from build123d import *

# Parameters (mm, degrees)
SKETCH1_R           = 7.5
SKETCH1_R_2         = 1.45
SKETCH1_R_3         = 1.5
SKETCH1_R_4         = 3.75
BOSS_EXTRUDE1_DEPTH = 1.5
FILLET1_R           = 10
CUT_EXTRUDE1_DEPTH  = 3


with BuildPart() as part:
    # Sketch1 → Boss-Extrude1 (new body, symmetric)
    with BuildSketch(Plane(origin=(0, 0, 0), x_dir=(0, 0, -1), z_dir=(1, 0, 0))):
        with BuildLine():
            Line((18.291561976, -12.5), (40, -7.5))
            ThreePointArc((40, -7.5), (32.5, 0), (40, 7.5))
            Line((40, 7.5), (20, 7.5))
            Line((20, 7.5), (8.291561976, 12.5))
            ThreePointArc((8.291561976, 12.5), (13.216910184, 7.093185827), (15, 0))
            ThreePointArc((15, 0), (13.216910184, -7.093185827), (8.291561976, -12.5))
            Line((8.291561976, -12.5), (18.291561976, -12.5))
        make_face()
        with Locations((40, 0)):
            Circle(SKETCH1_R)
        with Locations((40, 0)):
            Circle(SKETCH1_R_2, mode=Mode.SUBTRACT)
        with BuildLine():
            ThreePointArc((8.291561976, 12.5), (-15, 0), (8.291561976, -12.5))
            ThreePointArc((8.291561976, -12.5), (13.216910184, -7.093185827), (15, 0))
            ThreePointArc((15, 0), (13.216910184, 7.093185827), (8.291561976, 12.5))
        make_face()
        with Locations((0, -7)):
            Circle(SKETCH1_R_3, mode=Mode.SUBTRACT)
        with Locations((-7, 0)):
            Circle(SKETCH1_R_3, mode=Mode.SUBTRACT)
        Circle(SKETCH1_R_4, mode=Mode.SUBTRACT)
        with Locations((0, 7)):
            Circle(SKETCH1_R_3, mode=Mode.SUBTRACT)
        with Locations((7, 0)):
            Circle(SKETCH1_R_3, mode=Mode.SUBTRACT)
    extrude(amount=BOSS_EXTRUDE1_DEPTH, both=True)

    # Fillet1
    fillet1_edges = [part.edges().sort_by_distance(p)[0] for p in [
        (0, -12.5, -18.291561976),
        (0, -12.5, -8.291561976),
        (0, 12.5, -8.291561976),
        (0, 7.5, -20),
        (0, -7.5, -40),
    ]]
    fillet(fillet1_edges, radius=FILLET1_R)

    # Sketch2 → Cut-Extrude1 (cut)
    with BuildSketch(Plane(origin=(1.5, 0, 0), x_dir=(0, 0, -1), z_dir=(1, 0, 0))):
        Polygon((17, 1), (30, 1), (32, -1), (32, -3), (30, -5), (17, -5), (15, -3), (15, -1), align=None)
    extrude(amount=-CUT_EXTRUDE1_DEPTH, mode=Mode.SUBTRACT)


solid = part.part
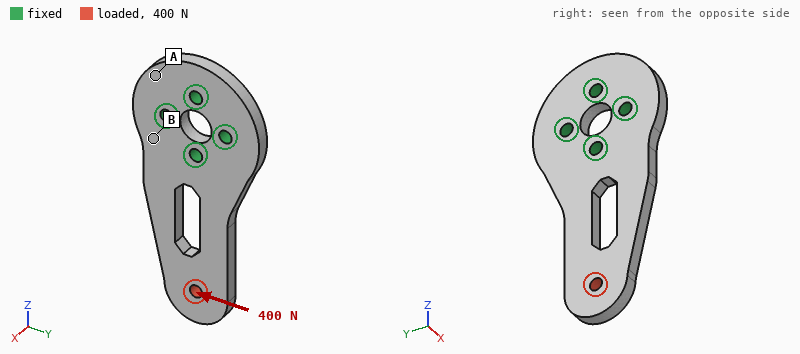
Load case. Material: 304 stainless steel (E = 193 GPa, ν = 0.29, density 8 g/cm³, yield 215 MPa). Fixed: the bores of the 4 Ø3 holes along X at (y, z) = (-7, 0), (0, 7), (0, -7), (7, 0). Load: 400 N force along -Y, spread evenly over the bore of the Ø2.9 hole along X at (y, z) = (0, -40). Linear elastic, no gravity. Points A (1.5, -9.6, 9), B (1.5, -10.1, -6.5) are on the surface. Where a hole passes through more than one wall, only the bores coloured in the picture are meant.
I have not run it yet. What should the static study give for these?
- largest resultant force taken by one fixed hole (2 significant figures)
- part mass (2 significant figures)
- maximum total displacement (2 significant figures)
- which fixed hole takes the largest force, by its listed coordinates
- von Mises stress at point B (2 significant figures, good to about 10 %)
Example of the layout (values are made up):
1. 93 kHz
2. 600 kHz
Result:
1. 690 N
2. 27 g
3. 29 µm
4. (-7, 0)
5. 34 MPa
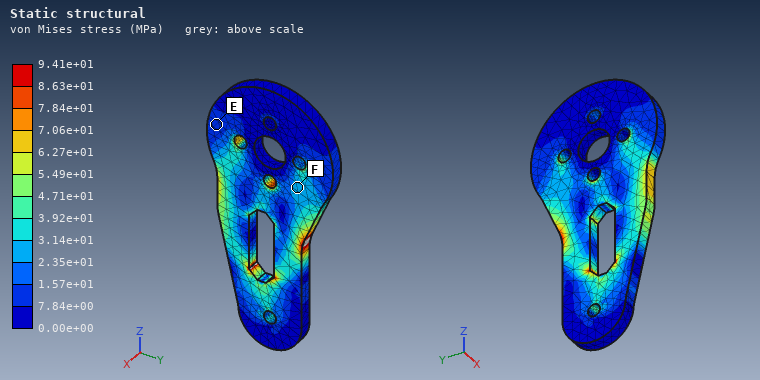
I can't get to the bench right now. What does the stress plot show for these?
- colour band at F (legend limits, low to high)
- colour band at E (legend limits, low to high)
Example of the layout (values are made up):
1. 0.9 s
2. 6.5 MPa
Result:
1. 2.35e+01 to 3.14e+01 MPa
2. 7.84e+00 to 1.57e+01 MPa
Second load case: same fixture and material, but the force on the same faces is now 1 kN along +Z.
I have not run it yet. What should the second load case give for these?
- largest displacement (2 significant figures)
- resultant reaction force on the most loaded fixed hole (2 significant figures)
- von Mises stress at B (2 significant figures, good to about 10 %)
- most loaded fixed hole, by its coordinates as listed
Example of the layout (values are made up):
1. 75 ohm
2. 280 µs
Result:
1. 5.6 µm
2. 430 N
3. 12 MPa
4. (0, -7)
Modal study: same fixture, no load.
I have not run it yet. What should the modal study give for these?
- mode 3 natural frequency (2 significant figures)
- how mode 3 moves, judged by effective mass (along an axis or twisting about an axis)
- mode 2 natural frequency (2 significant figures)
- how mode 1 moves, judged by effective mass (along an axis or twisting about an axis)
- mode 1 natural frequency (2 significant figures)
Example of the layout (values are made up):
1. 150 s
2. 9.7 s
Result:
1. 8400 Hz
2. along Y
3. 6600 Hz
4. along X
5. 1700 Hz
